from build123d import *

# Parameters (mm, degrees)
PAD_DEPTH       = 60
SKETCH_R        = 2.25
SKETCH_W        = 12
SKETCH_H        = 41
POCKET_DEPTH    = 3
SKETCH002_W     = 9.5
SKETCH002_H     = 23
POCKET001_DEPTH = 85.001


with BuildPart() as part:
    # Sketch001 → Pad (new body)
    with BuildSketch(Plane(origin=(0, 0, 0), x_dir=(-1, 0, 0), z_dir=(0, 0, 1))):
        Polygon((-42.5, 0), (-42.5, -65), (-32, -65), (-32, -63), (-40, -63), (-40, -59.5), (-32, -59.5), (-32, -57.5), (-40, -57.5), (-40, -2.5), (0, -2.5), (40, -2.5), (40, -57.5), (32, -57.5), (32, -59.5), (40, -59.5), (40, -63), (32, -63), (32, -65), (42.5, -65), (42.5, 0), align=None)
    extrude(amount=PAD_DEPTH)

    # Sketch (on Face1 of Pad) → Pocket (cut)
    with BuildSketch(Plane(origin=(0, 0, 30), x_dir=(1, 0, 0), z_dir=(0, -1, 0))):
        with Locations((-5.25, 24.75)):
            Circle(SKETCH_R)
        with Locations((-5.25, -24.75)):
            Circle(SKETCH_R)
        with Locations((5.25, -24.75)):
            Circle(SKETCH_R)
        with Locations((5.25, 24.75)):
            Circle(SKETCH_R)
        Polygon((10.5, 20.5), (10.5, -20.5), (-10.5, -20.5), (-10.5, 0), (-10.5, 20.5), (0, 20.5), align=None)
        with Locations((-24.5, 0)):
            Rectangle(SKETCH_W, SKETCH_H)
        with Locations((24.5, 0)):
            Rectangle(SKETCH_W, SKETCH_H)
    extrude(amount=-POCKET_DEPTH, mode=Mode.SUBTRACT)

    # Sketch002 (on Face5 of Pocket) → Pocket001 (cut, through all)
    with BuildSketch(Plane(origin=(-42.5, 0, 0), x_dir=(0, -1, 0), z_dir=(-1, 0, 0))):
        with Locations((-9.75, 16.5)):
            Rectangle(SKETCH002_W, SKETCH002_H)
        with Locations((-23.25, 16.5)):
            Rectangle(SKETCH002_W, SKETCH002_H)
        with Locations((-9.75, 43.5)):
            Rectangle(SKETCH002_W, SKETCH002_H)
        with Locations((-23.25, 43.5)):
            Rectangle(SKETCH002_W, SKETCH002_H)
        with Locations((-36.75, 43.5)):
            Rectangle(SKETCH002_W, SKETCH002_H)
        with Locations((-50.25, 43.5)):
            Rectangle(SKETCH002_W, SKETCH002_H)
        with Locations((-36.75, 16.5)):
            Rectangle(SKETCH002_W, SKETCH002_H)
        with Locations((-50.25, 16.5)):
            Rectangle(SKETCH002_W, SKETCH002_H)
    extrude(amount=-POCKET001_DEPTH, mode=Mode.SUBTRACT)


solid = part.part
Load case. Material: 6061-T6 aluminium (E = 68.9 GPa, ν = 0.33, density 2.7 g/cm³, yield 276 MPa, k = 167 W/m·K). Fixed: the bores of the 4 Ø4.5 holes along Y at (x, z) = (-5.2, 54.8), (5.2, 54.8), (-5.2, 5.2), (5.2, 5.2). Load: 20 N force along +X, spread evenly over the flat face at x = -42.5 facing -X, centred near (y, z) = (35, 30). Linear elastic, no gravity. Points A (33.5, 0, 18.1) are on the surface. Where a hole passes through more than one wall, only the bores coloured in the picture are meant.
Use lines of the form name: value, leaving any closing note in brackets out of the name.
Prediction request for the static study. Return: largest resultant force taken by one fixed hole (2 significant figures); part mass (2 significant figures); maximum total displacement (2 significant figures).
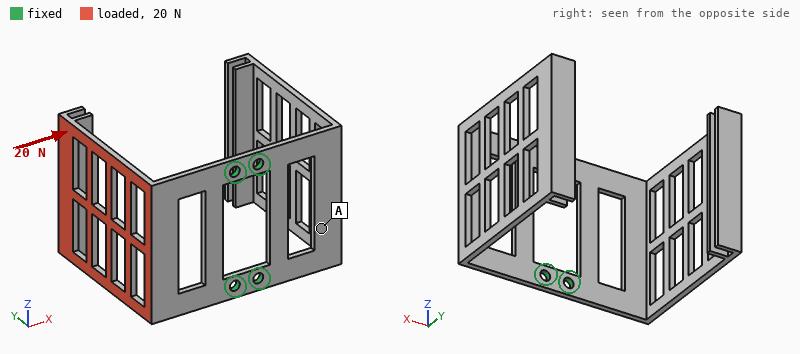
largest resultant force taken by one fixed hole: 9.4 N
part mass: 59 g
maximum total displacement: 1.3 mm
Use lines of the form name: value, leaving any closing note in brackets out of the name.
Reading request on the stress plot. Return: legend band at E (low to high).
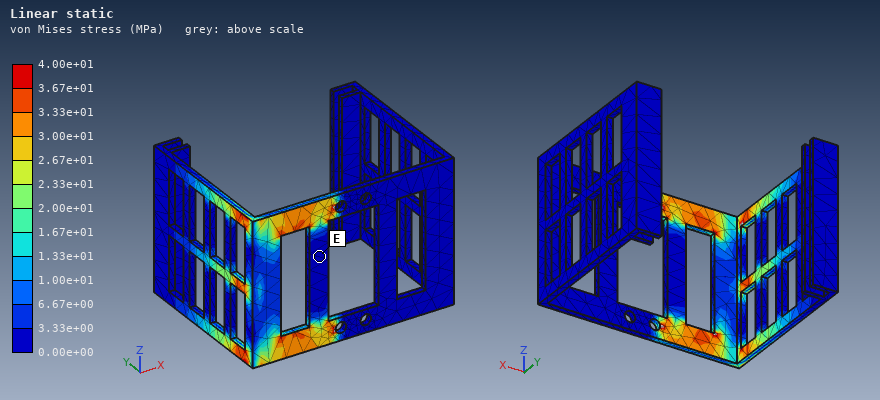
legend band at E: 0.00e+00 to 3.33e+00 MPa
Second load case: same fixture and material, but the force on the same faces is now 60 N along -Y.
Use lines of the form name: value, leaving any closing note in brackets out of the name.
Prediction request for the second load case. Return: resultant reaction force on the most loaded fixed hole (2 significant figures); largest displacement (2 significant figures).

resultant reaction force on the most loaded fixed hole: 31 N
largest displacement: 1.5 mm
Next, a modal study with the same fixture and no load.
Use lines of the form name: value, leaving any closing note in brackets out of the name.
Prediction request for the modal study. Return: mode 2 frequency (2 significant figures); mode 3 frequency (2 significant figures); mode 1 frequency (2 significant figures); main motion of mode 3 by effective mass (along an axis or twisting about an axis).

mode 2 frequency: 140 Hz
mode 3 frequency: 380 Hz
mode 1 frequency: 140 Hz
main motion of mode 3 by effective mass: along Z
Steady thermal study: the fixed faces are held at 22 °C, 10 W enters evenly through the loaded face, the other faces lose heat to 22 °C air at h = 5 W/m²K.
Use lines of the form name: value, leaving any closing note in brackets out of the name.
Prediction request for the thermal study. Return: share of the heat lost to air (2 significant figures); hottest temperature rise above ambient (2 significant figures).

share of the heat lost to air: 21 %
hottest temperature rise above ambient: 70 K
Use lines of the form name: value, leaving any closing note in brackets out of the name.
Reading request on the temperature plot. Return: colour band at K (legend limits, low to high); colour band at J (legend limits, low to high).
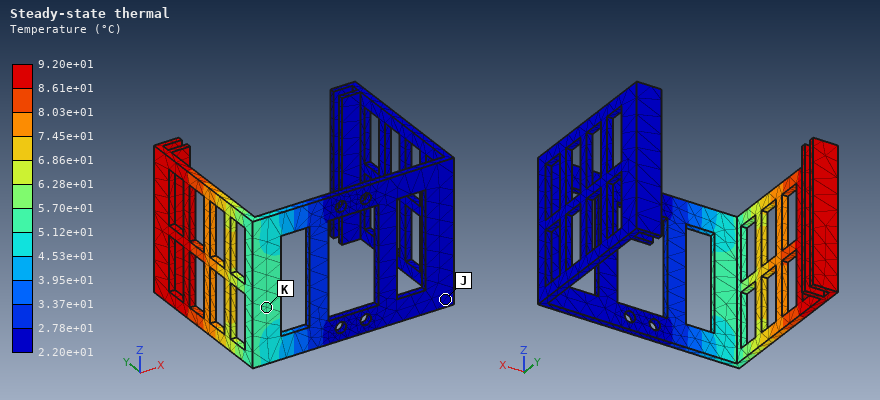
colour band at K: 5.12e+01 to 5.70e+01 °C
colour band at J: 2.20e+01 to 2.78e+01 °C
